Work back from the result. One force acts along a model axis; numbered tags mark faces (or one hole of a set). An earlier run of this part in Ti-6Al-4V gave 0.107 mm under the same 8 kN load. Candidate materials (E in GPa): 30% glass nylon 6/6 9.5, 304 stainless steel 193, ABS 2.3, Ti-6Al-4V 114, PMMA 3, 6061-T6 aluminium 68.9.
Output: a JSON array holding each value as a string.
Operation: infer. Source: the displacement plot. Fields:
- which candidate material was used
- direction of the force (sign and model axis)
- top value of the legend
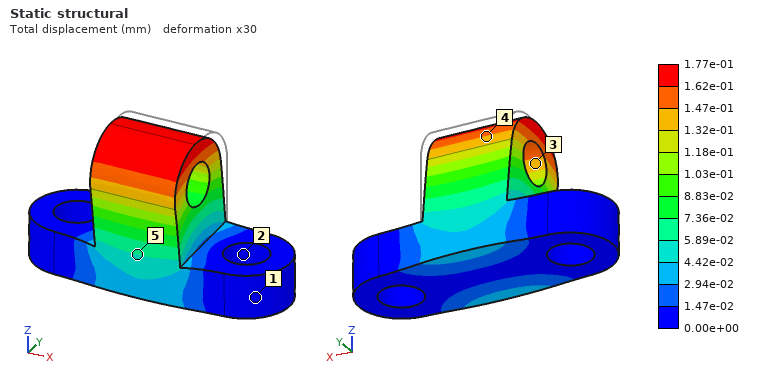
["6061-T6 aluminium", "-Y", "1.77e-01 mm"]
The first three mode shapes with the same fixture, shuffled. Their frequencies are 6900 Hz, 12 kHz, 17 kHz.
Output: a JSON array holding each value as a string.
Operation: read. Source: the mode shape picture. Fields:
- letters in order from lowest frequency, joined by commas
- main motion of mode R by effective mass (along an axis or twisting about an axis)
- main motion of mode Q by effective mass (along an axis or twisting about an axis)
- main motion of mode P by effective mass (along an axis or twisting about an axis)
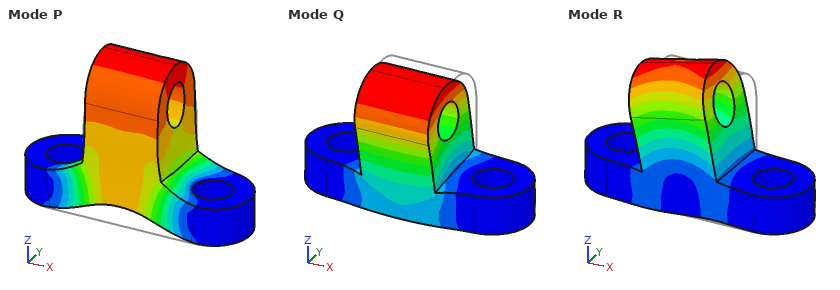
["Q, R, P", "along X", "along Y", "along Z"]
